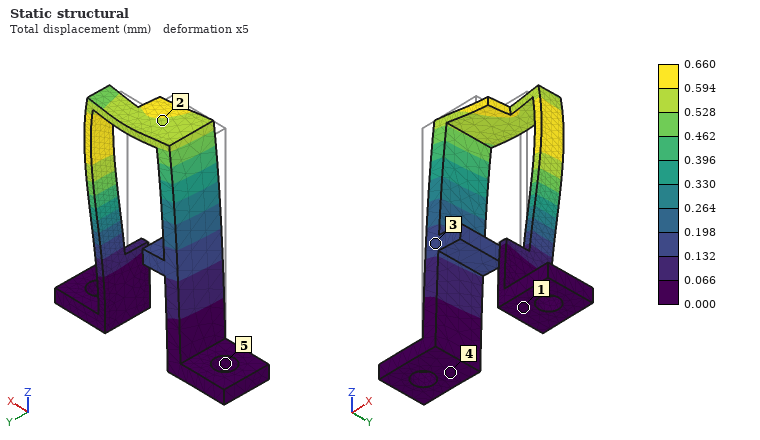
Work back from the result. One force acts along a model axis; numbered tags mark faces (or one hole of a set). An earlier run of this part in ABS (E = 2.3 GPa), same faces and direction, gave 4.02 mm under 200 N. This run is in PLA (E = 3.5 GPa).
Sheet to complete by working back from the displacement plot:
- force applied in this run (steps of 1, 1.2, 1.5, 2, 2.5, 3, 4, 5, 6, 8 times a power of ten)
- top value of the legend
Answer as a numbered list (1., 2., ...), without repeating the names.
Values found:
1. 50 N
2. 0.660 mm
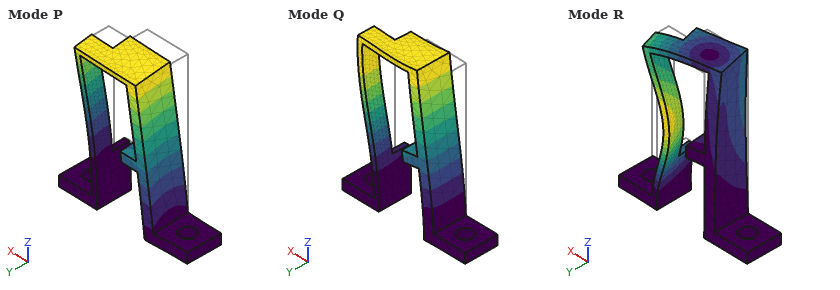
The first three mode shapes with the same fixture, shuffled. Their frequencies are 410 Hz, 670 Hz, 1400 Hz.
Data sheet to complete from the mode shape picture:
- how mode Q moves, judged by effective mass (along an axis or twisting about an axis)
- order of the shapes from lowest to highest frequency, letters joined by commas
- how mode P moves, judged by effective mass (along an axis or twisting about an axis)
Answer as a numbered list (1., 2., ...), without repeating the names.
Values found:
1. along X
2. Q, P, R
3. along Y
